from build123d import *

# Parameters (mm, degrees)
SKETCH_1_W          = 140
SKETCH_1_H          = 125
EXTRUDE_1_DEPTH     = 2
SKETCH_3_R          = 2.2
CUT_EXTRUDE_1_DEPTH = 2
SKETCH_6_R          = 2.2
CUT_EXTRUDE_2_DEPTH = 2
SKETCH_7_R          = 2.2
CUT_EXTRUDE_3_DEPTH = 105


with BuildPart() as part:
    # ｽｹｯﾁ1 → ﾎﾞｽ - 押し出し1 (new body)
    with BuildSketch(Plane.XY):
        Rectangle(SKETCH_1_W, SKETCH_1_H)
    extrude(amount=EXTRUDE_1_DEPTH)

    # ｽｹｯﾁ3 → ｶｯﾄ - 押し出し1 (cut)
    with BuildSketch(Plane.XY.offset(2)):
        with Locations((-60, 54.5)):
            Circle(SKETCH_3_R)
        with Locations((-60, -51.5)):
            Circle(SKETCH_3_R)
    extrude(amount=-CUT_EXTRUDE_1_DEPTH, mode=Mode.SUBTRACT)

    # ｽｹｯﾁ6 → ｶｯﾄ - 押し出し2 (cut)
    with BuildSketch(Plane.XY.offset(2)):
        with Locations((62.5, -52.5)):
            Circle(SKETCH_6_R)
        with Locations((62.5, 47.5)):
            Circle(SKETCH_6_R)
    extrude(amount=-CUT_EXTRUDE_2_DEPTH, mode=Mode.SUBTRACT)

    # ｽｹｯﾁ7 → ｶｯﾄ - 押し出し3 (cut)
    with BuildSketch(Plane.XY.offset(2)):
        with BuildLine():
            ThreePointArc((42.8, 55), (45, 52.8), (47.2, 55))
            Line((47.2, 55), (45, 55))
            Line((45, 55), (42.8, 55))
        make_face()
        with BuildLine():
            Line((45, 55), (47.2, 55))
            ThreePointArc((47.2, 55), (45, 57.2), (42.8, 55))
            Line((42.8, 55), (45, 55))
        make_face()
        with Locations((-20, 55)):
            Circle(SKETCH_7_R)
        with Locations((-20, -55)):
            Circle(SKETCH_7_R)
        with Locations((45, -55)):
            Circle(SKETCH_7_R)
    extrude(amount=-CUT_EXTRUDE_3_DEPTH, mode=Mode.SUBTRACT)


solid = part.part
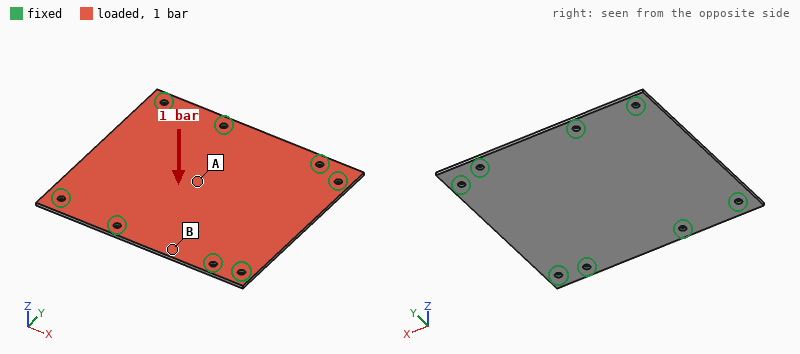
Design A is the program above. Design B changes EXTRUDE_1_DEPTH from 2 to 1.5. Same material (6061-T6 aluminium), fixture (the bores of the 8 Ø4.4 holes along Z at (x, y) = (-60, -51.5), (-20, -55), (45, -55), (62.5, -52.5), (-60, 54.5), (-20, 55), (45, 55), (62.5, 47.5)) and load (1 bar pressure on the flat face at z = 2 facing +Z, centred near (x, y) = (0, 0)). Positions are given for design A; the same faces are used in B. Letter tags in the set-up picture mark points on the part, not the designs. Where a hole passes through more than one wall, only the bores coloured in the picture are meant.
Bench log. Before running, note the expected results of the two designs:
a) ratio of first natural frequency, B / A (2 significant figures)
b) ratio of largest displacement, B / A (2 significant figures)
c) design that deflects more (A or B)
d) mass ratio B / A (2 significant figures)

0.76
2.3
B
0.75
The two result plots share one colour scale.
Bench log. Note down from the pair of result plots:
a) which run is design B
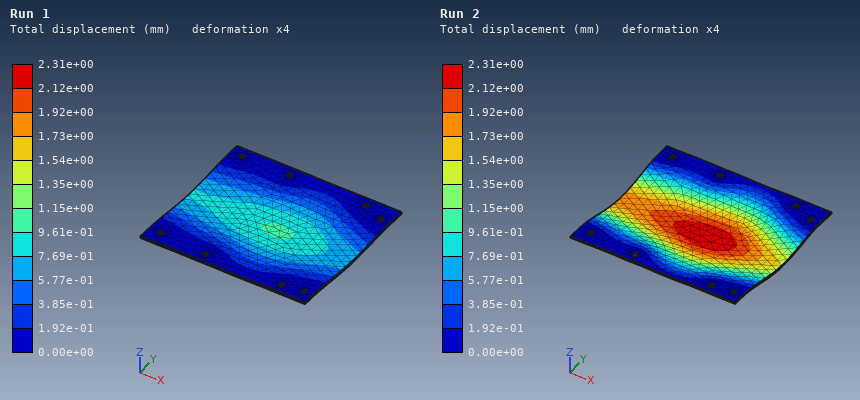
Run 2
